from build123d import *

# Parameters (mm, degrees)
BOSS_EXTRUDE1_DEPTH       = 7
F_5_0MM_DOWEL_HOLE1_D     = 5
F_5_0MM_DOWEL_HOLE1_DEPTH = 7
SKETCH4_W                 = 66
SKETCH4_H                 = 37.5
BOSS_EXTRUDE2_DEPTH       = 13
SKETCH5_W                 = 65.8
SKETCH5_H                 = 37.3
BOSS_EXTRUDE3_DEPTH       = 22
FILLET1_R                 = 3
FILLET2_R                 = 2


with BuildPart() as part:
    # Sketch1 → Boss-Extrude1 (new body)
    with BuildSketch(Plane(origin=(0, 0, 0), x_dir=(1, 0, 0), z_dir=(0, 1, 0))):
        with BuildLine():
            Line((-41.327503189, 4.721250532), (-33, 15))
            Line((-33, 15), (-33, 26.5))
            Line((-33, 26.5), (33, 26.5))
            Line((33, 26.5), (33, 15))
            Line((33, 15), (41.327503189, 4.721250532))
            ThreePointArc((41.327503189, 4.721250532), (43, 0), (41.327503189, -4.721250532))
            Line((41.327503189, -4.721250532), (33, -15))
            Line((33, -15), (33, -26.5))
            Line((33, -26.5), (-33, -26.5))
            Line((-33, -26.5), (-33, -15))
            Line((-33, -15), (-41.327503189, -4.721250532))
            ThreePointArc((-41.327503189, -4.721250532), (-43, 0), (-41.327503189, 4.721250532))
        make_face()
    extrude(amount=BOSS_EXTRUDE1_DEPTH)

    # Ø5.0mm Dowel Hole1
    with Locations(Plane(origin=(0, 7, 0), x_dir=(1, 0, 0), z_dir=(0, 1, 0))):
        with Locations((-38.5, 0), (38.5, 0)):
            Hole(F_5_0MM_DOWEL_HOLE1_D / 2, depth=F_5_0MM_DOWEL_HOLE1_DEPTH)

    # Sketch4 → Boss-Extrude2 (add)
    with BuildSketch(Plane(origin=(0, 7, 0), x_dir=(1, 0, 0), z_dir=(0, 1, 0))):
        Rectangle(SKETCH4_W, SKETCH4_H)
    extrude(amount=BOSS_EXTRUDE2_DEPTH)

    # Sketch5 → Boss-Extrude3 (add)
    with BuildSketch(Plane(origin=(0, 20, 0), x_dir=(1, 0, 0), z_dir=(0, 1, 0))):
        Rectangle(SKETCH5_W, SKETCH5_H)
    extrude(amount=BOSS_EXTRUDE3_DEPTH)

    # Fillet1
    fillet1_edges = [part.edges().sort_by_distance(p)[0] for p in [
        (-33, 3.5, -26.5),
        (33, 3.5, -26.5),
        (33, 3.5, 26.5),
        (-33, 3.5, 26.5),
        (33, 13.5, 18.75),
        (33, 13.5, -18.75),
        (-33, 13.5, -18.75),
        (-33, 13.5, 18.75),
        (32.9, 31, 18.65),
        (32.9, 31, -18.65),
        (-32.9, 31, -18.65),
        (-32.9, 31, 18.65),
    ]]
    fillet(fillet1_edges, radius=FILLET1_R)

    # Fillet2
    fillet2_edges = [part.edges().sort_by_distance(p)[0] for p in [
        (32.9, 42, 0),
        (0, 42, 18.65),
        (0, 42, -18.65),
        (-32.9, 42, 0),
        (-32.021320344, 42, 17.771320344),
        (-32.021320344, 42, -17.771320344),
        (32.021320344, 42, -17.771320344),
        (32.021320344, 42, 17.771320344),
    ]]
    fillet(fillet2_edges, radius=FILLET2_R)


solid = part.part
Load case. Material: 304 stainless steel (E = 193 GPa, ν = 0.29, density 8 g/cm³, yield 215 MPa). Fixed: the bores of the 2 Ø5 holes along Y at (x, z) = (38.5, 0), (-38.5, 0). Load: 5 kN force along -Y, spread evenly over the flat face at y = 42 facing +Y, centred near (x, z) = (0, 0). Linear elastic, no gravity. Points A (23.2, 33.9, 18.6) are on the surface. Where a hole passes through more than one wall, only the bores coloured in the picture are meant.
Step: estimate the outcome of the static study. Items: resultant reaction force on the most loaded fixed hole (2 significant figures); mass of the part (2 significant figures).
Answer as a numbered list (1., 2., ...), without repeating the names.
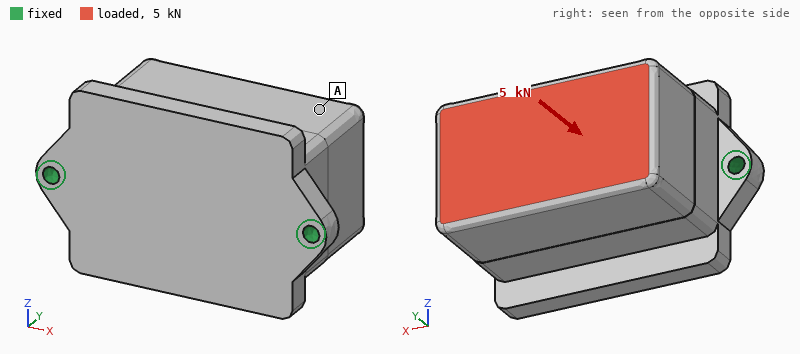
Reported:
1. 2.7 kN
2. 900 g
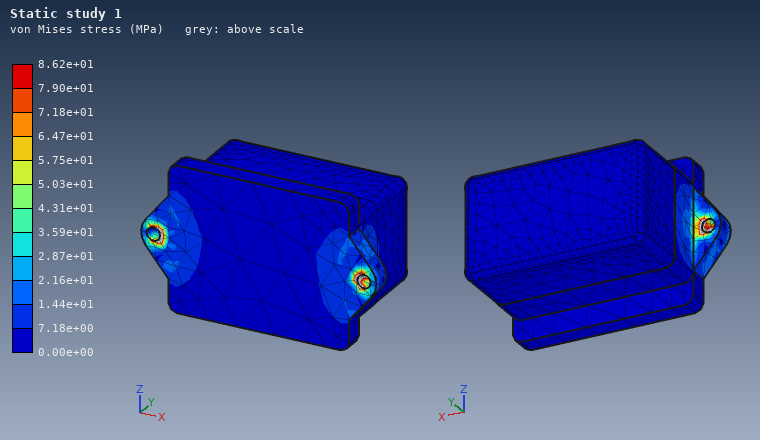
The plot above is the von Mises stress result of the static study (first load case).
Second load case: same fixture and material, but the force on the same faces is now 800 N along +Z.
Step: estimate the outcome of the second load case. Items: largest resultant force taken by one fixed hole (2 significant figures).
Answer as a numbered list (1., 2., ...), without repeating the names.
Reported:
1. 400 N
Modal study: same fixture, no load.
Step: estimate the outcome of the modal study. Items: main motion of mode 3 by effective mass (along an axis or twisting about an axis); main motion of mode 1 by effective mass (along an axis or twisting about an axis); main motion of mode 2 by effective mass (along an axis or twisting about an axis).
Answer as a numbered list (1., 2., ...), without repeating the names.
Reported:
1. along X
2. along Z
3. along Y
